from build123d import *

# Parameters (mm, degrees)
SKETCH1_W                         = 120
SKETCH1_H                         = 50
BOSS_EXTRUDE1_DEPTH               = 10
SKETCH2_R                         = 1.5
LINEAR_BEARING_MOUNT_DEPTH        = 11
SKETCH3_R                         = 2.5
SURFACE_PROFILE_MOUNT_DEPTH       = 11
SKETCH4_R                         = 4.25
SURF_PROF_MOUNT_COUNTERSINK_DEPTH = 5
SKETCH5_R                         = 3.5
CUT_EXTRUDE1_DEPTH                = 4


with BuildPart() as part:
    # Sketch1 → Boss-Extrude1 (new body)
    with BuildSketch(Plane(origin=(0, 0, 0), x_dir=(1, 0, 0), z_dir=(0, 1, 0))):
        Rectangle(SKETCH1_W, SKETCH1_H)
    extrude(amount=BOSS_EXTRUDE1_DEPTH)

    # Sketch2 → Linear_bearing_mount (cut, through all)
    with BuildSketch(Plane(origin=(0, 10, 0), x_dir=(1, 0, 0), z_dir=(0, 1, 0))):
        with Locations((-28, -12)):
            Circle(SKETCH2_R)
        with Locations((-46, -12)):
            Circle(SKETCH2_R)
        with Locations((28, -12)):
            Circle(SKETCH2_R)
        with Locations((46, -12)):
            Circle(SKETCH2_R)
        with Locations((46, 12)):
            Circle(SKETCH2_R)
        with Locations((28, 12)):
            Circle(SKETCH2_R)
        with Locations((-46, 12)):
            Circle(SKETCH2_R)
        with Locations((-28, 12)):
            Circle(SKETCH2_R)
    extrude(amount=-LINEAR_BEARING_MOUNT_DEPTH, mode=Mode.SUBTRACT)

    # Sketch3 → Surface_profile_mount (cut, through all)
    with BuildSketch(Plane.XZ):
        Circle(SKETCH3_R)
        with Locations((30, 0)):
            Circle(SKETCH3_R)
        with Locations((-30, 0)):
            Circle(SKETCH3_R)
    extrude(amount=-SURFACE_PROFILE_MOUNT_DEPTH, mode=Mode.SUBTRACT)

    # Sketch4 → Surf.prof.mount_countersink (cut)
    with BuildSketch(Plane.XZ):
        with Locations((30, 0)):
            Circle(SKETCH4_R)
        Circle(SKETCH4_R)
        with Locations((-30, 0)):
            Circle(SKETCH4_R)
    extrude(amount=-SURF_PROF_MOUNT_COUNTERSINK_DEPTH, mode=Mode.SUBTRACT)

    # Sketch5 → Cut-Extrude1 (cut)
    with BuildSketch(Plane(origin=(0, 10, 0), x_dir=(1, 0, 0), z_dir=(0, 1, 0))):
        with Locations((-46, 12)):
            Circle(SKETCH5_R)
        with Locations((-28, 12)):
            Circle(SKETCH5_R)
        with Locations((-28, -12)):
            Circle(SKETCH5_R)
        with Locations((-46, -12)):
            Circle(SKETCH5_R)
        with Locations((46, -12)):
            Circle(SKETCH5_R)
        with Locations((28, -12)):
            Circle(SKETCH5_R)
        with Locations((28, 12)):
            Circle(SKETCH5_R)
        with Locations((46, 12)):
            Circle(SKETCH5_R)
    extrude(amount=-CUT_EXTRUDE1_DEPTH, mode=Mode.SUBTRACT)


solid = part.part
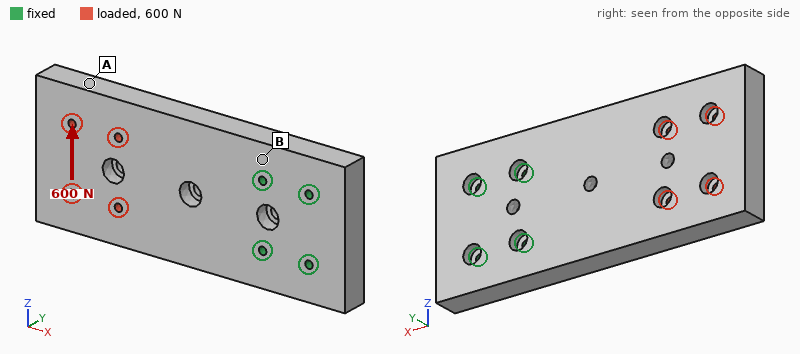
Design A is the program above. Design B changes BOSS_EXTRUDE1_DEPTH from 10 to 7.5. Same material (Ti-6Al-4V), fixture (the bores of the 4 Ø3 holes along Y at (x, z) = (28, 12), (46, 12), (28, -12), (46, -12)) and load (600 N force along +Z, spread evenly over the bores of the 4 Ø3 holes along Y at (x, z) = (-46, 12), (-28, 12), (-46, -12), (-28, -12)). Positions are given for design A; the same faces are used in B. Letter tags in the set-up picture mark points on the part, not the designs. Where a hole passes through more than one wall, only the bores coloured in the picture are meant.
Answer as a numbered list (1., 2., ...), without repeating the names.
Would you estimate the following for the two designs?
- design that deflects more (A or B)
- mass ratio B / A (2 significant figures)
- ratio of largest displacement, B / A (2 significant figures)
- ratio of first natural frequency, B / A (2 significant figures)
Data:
1. B
2. 0.75
3. 1.2
4. 0.79
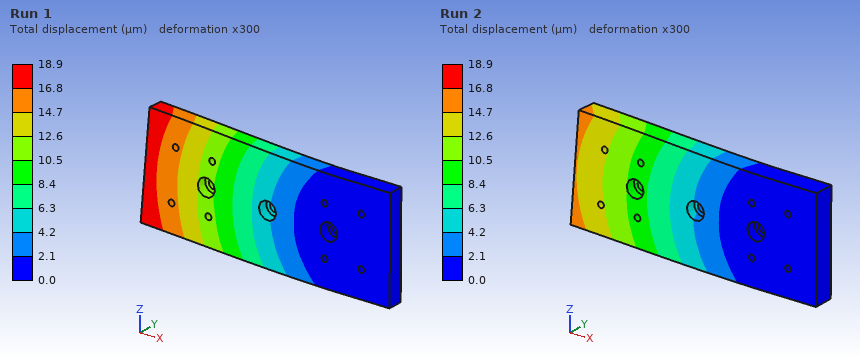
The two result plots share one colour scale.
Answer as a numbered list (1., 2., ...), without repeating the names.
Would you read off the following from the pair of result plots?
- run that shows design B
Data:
1. Run 1
